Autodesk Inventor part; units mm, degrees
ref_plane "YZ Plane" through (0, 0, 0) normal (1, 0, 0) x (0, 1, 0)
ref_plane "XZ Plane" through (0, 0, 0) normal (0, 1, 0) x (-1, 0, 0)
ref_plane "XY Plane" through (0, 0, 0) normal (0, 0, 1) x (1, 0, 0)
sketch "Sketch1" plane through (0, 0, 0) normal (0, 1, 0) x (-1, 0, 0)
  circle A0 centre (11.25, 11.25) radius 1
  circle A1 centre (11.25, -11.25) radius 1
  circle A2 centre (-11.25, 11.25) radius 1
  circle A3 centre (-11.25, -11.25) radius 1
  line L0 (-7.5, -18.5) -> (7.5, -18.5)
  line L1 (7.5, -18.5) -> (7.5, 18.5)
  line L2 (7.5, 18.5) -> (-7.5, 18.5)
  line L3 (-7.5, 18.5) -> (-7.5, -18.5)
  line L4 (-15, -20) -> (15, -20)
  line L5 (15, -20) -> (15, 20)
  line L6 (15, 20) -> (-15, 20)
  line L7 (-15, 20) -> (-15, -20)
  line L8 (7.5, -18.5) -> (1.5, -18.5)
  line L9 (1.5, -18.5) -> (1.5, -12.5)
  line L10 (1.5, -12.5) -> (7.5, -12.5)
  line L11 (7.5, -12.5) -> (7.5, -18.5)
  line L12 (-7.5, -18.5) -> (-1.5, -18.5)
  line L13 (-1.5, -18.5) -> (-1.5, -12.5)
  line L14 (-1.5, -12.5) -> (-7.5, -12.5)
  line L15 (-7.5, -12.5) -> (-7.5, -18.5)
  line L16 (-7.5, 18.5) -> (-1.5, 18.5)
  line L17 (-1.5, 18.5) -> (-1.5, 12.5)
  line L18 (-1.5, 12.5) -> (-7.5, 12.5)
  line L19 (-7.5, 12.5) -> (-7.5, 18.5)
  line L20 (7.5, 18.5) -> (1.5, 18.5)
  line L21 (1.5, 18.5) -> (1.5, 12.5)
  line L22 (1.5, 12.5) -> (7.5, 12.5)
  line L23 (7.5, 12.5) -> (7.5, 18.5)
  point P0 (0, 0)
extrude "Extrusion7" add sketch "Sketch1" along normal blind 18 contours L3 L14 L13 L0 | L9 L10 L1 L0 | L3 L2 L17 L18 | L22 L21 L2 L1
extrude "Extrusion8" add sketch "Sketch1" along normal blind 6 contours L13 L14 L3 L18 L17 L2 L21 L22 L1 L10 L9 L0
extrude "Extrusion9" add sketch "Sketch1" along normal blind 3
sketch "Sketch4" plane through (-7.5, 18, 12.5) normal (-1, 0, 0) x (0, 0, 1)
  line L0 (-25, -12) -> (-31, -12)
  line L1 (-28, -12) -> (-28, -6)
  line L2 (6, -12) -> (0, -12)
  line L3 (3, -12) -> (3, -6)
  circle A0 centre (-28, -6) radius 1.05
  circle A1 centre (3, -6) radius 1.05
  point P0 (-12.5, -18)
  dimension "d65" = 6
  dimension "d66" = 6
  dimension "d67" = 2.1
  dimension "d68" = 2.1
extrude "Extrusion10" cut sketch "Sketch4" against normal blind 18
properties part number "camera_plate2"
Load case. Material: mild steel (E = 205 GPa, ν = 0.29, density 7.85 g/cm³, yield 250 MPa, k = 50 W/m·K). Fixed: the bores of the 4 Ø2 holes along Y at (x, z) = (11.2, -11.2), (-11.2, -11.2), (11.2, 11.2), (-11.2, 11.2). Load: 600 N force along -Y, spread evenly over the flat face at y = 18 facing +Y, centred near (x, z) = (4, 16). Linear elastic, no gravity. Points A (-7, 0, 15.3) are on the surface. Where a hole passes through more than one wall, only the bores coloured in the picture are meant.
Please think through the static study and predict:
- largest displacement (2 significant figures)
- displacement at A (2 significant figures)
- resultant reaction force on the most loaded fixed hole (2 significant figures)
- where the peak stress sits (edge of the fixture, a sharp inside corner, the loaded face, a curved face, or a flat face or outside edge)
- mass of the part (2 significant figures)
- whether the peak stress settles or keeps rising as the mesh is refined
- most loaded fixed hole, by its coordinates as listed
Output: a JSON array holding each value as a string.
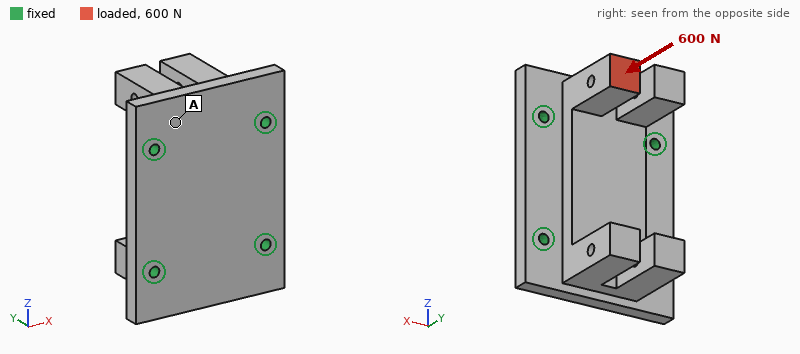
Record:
["9.5 µm", "2.3 µm", "490 N", "edge of the fixture", "54 g", "keeps rising", "(11.2, 11.2)"]
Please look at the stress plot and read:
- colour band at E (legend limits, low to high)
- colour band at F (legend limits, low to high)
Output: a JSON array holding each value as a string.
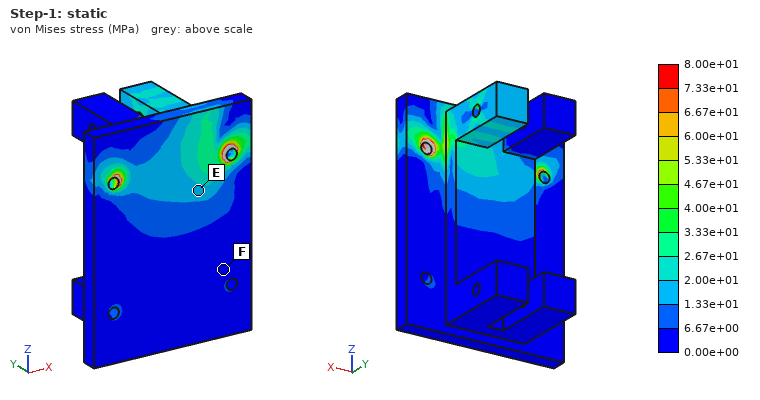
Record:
["1.33e+01 to 2.00e+01 MPa", "0.00e+00 to 6.67e+00 MPa"]
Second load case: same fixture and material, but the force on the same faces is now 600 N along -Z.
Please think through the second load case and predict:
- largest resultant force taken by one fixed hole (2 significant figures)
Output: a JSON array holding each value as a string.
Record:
["350 N"]
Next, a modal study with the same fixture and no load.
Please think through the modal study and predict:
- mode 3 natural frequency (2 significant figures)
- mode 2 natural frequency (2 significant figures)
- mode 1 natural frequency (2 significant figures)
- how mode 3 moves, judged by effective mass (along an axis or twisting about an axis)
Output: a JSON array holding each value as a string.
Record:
["17 kHz", "12 kHz", "12 kHz", "along X"]
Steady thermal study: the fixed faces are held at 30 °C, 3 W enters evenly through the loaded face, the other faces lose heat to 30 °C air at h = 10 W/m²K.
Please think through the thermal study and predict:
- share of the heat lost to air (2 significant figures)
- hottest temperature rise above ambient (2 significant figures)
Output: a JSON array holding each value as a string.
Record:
["4.4 %", "31 K"]
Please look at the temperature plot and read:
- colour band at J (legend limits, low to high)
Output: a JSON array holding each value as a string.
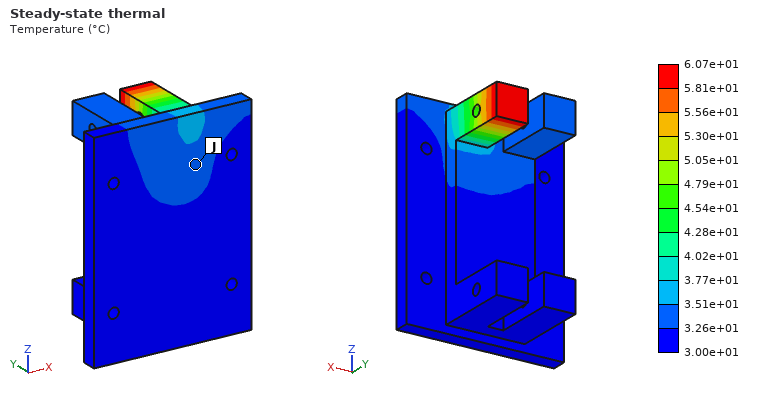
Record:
["3.26e+01 to 3.51e+01 °C"]
